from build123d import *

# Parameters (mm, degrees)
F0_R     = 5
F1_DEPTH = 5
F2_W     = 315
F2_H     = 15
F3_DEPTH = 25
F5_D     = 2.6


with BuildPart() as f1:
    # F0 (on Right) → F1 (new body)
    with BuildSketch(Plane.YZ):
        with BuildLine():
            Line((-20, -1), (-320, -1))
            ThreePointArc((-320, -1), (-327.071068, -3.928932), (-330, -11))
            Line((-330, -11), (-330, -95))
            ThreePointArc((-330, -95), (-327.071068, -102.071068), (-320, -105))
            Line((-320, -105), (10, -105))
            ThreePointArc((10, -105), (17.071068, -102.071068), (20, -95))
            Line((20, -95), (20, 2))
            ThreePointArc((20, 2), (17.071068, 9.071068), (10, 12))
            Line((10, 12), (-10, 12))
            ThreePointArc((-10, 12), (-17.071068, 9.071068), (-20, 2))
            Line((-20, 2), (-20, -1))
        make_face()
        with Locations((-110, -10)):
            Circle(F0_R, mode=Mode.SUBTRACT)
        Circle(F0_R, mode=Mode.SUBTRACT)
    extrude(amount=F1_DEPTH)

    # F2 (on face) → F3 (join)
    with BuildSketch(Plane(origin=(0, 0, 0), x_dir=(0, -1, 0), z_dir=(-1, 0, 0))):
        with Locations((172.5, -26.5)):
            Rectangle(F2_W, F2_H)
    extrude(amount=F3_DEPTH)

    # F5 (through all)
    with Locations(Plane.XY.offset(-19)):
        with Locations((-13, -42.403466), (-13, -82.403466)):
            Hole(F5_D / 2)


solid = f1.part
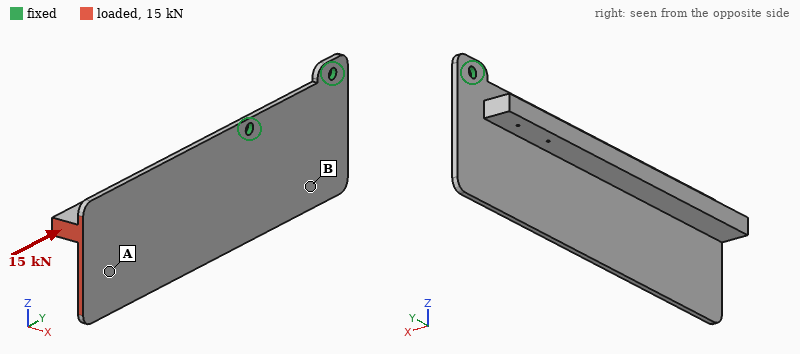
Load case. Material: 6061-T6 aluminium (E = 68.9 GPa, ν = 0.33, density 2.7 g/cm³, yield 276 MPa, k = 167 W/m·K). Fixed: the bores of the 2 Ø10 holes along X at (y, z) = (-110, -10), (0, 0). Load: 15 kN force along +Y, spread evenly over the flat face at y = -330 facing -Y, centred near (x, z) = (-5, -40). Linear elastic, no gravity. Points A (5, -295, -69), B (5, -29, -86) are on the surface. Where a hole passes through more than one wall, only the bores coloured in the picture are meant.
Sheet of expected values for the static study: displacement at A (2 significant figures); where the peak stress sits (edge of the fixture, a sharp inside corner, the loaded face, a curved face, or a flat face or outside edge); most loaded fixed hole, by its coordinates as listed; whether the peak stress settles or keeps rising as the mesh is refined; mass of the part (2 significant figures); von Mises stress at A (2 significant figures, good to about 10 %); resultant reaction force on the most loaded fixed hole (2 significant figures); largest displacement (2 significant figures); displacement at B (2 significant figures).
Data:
0.33 mm
edge of the fixture
(-110, -10)
keeps rising
810 g
18 MPa
11 kN
0.43 mm
0.14 mm
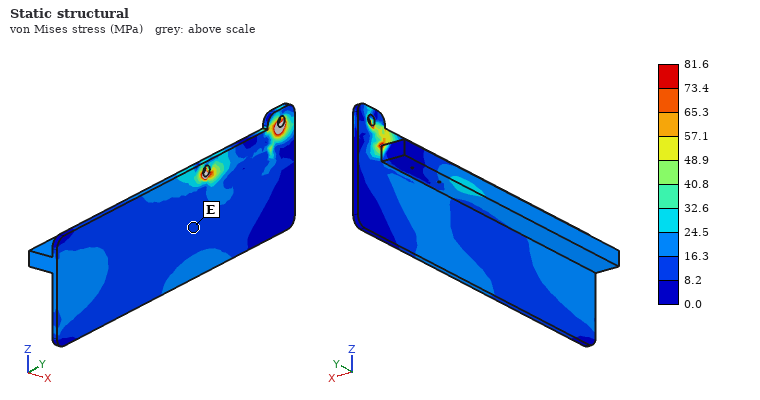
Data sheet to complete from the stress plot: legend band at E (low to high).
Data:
8.2 to 16.3 MPa
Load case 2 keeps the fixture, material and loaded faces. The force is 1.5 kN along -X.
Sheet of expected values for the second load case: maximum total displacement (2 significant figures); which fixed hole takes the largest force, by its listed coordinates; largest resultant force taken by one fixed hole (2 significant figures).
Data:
3.9 mm
(-110, -10)
5.6 kN
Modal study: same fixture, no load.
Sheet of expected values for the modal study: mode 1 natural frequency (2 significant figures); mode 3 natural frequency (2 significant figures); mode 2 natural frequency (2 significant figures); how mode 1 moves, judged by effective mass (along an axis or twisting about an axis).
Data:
260 Hz
680 Hz
370 Hz
along X
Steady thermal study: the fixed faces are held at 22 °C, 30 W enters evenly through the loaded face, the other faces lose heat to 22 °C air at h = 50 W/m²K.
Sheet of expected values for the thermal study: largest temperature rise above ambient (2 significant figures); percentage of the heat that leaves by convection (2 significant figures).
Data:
22 K
85 %
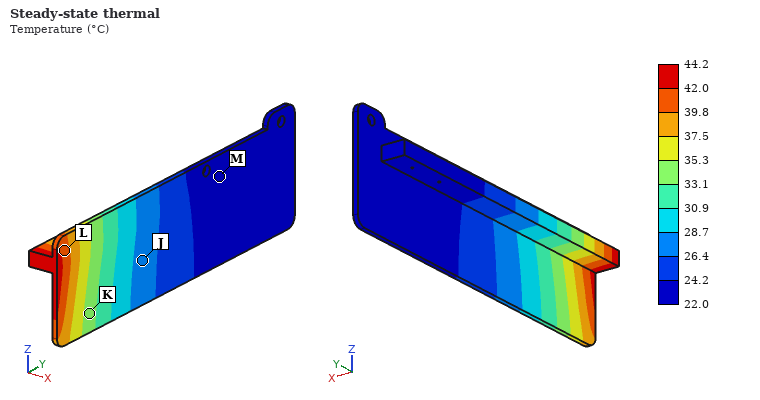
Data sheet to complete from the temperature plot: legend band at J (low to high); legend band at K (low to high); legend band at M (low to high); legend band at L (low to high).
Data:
26.4 to 28.7 °C
33.1 to 35.3 °C
22.0 to 24.2 °C
39.8 to 42.0 °C
